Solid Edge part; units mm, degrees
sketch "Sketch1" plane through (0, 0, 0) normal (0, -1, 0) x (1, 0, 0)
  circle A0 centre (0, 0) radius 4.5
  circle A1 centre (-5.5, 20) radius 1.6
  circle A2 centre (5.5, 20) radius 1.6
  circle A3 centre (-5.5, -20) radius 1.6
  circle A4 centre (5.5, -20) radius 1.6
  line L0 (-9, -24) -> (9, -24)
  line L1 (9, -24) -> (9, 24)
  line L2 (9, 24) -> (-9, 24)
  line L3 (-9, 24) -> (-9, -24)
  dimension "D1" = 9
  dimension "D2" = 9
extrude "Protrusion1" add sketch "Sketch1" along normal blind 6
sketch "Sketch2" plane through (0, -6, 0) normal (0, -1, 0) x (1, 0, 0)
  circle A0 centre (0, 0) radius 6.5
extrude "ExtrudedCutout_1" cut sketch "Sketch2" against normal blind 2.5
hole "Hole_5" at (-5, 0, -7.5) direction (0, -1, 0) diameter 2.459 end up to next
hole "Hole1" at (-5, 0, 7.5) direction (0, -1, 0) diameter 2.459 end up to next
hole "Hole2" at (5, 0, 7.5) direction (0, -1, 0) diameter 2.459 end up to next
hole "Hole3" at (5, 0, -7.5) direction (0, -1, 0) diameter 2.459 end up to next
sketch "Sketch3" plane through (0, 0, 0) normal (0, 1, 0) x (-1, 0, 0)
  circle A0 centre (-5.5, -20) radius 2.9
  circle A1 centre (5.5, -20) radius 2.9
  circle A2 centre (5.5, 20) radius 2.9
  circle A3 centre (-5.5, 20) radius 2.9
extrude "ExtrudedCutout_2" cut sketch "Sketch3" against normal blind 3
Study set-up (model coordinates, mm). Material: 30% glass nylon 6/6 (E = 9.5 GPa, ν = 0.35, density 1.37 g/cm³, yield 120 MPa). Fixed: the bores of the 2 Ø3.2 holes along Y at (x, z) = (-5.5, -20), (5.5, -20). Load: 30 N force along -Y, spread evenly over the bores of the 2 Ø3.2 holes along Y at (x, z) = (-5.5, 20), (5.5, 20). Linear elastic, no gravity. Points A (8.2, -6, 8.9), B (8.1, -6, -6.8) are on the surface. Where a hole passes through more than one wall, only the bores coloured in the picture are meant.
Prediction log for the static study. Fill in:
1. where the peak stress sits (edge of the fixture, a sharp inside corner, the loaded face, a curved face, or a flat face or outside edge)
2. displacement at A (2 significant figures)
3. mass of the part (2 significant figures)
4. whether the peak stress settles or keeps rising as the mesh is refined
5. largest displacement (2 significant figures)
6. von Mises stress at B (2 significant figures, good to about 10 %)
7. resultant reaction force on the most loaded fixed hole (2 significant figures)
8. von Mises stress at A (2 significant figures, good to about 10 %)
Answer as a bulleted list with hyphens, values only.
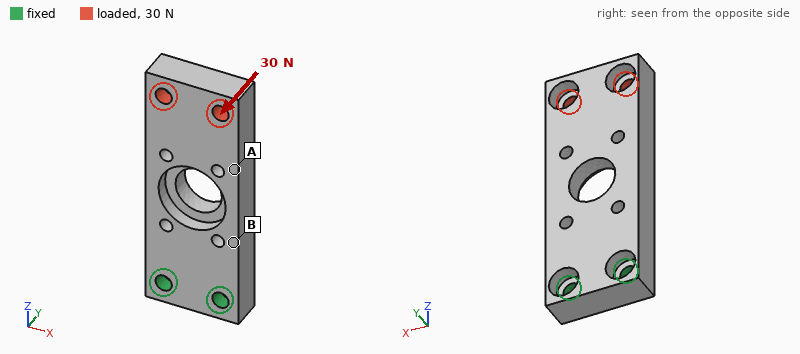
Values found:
- edge of the fixture
- 0.26 mm
- 5.6 g
- keeps rising
- 0.49 mm
- 15 MPa
- 18 N
- 5.7 MPa
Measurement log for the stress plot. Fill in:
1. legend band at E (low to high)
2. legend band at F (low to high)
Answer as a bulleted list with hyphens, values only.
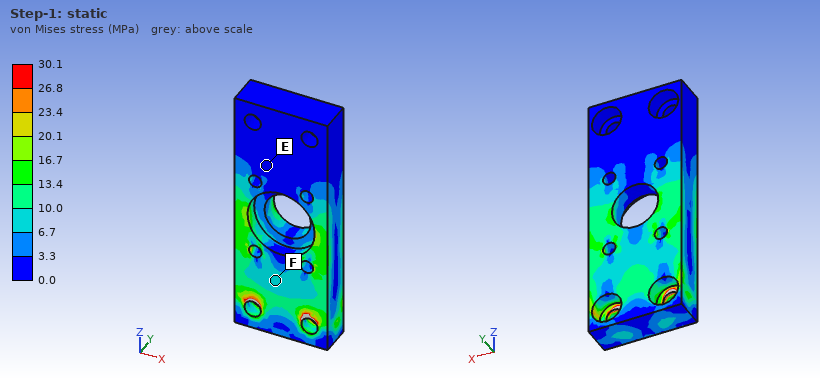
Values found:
- 0.0 to 3.3 MPa
- 6.7 to 10.0 MPa
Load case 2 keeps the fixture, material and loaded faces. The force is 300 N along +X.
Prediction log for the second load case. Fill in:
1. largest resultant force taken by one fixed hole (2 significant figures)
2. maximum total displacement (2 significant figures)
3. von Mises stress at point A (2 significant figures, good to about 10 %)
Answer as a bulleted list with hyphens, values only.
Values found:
- 940 N
- 0.55 mm
- 14 MPa
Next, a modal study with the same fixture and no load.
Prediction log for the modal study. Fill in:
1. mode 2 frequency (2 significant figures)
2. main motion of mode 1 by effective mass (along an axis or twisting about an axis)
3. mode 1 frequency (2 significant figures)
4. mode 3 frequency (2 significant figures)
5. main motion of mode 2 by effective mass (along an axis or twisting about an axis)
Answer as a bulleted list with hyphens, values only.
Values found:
- 3000 Hz
- along Y
- 1000 Hz
- 4600 Hz
- along X
